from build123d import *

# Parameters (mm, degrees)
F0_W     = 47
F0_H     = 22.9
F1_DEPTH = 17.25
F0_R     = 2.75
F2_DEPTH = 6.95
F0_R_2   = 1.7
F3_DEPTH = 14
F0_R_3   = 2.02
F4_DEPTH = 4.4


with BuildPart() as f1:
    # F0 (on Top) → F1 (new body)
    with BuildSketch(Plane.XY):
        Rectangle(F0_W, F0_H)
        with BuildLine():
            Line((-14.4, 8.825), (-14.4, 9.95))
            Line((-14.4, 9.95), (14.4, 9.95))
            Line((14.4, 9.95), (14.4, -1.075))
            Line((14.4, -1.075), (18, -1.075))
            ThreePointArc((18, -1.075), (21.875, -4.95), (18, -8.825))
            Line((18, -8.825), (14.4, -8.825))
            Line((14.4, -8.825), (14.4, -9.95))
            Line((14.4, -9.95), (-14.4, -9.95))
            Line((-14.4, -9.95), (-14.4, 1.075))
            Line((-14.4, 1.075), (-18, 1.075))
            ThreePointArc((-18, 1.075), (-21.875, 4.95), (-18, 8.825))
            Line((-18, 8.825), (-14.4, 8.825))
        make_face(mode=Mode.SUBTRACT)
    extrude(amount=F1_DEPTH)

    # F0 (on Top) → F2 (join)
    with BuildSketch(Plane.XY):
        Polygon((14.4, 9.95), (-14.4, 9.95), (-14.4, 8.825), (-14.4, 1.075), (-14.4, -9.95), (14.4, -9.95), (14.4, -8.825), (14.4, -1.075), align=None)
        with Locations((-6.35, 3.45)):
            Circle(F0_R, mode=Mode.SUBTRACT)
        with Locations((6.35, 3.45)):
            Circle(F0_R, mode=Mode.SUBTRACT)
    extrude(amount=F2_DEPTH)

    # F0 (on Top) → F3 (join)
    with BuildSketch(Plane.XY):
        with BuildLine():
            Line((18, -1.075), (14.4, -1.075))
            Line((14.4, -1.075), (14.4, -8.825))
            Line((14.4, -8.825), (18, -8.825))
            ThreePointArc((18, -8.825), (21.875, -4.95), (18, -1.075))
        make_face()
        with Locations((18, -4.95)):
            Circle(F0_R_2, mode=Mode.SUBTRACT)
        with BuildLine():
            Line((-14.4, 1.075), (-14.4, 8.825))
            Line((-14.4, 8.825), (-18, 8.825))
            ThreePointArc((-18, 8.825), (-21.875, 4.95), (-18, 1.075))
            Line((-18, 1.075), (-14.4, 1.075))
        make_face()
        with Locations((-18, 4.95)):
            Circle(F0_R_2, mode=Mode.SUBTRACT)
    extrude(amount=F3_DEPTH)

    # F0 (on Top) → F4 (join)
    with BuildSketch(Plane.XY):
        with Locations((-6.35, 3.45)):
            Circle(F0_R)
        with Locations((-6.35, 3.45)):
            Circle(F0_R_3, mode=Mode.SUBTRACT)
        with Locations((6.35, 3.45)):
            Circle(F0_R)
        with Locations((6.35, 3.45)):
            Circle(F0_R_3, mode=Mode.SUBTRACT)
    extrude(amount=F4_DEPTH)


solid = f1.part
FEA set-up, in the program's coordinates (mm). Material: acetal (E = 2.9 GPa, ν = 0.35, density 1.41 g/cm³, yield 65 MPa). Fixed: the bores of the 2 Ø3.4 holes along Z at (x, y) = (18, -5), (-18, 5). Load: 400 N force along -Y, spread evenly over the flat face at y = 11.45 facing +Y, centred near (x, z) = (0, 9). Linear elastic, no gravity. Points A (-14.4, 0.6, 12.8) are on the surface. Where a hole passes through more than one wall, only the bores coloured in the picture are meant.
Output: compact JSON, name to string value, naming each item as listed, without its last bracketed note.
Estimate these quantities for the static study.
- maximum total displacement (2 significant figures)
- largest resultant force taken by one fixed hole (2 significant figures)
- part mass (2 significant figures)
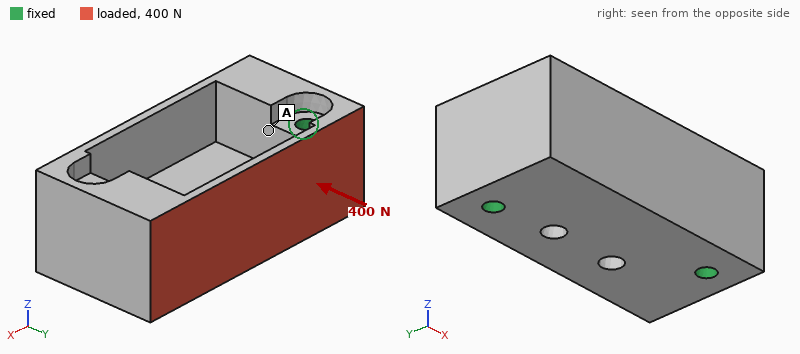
{"maximum total displacement": "0.60 mm", "largest resultant force taken by one fixed hole": "210 N", "part mass": "17 g"}
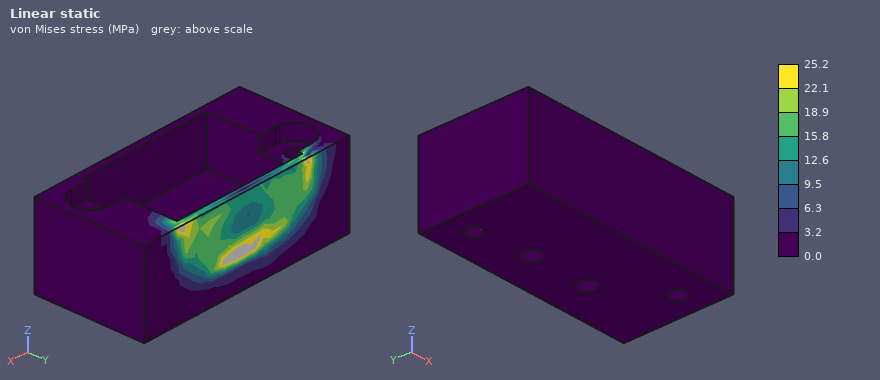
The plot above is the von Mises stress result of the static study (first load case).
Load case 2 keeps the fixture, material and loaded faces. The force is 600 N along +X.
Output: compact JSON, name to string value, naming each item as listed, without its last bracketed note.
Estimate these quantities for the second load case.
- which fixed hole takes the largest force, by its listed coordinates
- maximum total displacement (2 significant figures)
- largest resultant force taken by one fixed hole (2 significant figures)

{"which fixed hole takes the largest force, by its listed coordinates": "(-18, 5)", "maximum total displacement": "65 µm", "largest resultant force taken by one fixed hole": "430 N"}
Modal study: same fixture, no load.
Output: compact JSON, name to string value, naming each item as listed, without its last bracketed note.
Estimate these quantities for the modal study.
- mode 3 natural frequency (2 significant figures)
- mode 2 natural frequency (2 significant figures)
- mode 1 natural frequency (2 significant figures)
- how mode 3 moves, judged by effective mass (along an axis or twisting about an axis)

{"mode 3 natural frequency": "6200 Hz", "mode 2 natural frequency": "4400 Hz", "mode 1 natural frequency": "4300 Hz", "how mode 3 moves, judged by effective mass": "along Z"}
